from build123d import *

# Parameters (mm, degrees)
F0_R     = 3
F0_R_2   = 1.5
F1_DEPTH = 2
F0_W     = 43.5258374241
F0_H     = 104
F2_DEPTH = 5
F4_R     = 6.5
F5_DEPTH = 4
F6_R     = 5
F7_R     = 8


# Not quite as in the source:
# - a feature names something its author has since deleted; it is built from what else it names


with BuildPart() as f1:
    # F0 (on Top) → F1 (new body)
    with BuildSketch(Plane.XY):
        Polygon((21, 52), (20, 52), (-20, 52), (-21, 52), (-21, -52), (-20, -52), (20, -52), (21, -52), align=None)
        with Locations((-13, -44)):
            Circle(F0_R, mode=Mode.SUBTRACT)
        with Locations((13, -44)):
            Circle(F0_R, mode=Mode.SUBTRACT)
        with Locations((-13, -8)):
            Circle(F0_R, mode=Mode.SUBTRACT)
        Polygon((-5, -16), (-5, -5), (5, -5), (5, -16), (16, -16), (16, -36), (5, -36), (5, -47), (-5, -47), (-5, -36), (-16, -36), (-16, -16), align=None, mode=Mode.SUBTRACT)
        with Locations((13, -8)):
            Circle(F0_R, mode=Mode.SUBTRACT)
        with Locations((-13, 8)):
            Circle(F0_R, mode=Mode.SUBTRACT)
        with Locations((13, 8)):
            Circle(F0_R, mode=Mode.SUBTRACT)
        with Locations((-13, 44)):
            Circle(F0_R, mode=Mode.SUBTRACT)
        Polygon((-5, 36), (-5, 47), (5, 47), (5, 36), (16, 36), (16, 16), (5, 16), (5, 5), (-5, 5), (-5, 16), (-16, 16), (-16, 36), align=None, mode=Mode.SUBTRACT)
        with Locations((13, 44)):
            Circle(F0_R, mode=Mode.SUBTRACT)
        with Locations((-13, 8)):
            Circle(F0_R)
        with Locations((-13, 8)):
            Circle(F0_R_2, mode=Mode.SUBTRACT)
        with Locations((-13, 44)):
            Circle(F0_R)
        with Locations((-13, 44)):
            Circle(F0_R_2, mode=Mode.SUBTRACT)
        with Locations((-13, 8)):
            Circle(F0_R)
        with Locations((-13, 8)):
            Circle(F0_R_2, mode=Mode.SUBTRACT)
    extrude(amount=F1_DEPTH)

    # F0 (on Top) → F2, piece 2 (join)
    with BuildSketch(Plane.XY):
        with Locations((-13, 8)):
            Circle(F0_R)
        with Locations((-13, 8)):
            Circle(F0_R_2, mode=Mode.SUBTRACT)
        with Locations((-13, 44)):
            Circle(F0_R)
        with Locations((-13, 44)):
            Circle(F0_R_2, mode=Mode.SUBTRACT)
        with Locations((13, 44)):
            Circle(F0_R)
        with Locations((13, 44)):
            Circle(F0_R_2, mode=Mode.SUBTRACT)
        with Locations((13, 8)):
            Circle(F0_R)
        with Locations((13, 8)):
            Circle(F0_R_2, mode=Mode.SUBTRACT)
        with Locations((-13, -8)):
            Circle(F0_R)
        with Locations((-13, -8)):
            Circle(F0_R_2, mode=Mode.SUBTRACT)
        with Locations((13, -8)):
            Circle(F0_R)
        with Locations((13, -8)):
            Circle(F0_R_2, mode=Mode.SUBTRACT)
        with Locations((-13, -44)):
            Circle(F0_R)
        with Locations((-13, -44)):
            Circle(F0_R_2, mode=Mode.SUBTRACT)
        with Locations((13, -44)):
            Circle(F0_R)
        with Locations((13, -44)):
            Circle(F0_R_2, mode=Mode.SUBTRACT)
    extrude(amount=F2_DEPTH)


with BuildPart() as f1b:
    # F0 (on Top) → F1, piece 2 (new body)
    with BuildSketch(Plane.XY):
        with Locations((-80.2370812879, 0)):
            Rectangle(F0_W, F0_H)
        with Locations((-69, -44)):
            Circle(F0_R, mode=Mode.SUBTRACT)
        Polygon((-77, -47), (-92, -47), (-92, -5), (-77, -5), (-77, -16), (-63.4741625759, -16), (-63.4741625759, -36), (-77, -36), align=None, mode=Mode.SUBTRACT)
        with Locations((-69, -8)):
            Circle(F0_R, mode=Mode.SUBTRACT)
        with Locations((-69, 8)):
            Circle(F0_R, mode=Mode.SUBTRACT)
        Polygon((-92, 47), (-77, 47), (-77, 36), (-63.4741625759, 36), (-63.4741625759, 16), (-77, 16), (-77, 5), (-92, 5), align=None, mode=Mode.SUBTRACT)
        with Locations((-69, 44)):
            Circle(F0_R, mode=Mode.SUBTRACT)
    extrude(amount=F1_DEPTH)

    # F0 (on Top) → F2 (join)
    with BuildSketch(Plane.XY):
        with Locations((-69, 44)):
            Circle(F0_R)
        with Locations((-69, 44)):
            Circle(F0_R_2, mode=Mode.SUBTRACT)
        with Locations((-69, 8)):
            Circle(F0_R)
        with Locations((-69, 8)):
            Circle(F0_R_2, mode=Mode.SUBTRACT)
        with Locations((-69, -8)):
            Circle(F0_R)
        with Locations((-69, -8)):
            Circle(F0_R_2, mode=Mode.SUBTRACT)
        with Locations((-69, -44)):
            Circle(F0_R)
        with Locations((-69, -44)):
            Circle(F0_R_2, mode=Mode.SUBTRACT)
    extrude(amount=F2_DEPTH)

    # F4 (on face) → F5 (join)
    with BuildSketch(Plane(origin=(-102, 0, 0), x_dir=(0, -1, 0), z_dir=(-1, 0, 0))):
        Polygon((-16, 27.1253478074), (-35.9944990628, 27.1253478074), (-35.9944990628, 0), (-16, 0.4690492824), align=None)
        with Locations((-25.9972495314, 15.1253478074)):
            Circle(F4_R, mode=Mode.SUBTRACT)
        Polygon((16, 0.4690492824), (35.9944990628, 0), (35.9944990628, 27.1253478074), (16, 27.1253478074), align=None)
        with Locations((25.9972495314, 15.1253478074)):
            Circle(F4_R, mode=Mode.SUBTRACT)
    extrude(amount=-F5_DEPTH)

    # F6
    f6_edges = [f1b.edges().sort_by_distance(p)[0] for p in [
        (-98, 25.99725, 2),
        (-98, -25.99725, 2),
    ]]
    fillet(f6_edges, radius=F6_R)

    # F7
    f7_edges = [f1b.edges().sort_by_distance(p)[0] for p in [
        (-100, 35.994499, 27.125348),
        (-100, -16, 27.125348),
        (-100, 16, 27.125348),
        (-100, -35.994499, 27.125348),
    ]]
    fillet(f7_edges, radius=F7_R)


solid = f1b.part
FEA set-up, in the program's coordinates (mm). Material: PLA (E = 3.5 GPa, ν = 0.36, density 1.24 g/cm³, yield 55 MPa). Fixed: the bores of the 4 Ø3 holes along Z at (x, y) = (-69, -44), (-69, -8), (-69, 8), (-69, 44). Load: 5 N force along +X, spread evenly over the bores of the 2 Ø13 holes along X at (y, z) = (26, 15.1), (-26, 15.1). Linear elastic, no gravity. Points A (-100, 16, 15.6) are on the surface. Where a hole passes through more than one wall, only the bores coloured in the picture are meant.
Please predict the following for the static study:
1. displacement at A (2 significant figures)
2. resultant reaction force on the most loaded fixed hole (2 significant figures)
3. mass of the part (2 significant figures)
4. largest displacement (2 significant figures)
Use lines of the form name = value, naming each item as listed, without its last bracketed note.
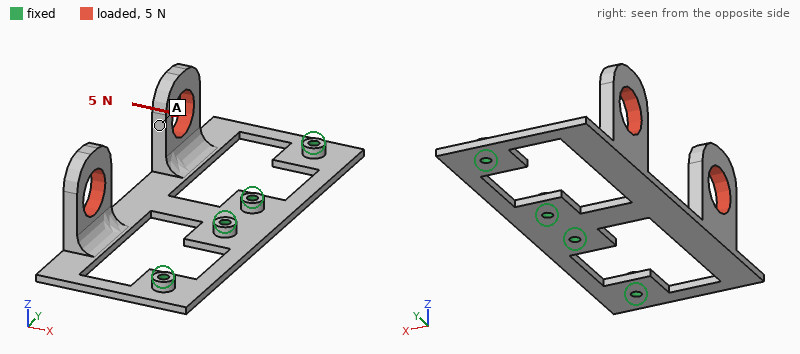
displacement at A = 0.82 mm
resultant reaction force on the most loaded fixed hole = 1.6 N
mass of the part = 11 g
largest displacement = 1.2 mm
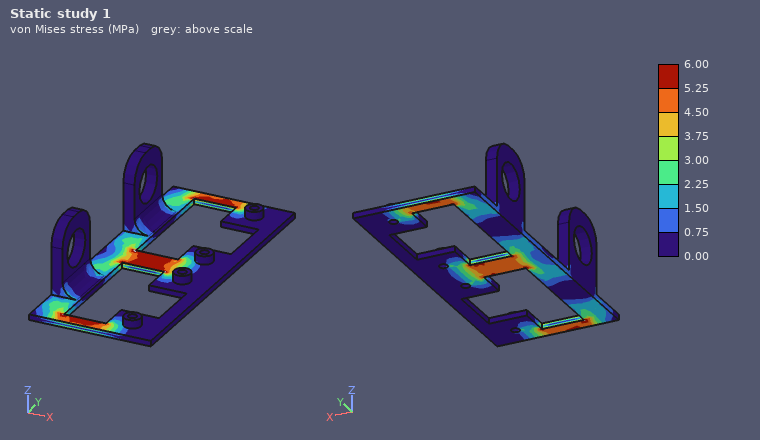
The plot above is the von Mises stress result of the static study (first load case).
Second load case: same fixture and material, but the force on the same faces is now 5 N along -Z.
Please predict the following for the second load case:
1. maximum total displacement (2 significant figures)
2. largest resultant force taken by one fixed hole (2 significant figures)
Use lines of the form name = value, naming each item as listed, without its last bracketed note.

maximum total displacement = 1.4 mm
largest resultant force taken by one fixed hole = 1.4 N
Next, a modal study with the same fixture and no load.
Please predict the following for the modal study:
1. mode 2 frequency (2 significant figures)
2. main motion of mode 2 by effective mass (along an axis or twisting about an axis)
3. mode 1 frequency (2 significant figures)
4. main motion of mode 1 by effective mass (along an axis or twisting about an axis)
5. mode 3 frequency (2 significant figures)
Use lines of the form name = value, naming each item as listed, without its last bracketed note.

mode 2 frequency = 260 Hz
main motion of mode 2 by effective mass = twisting about X
mode 1 frequency = 150 Hz
main motion of mode 1 by effective mass = along Z
mode 3 frequency = 480 Hz
